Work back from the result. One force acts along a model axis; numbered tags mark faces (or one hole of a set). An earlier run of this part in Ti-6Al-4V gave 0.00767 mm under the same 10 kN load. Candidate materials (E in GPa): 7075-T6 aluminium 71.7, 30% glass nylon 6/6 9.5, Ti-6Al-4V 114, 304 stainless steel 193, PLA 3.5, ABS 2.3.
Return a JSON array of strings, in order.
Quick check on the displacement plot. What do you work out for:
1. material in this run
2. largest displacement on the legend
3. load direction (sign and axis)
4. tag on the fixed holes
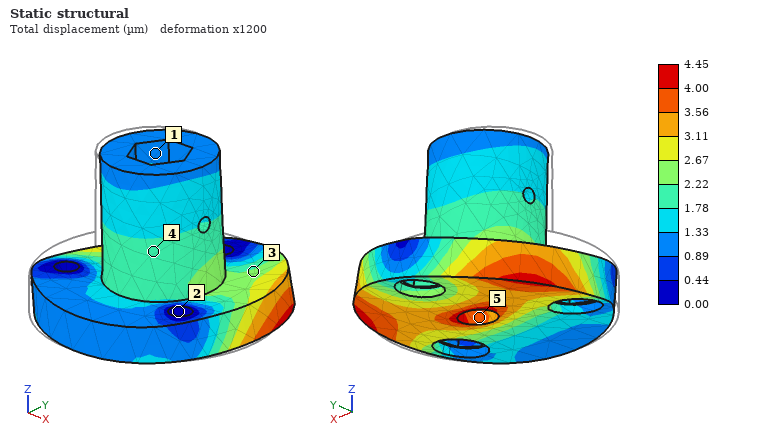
["304 stainless steel", "4.45 µm", "+X", "2"]
